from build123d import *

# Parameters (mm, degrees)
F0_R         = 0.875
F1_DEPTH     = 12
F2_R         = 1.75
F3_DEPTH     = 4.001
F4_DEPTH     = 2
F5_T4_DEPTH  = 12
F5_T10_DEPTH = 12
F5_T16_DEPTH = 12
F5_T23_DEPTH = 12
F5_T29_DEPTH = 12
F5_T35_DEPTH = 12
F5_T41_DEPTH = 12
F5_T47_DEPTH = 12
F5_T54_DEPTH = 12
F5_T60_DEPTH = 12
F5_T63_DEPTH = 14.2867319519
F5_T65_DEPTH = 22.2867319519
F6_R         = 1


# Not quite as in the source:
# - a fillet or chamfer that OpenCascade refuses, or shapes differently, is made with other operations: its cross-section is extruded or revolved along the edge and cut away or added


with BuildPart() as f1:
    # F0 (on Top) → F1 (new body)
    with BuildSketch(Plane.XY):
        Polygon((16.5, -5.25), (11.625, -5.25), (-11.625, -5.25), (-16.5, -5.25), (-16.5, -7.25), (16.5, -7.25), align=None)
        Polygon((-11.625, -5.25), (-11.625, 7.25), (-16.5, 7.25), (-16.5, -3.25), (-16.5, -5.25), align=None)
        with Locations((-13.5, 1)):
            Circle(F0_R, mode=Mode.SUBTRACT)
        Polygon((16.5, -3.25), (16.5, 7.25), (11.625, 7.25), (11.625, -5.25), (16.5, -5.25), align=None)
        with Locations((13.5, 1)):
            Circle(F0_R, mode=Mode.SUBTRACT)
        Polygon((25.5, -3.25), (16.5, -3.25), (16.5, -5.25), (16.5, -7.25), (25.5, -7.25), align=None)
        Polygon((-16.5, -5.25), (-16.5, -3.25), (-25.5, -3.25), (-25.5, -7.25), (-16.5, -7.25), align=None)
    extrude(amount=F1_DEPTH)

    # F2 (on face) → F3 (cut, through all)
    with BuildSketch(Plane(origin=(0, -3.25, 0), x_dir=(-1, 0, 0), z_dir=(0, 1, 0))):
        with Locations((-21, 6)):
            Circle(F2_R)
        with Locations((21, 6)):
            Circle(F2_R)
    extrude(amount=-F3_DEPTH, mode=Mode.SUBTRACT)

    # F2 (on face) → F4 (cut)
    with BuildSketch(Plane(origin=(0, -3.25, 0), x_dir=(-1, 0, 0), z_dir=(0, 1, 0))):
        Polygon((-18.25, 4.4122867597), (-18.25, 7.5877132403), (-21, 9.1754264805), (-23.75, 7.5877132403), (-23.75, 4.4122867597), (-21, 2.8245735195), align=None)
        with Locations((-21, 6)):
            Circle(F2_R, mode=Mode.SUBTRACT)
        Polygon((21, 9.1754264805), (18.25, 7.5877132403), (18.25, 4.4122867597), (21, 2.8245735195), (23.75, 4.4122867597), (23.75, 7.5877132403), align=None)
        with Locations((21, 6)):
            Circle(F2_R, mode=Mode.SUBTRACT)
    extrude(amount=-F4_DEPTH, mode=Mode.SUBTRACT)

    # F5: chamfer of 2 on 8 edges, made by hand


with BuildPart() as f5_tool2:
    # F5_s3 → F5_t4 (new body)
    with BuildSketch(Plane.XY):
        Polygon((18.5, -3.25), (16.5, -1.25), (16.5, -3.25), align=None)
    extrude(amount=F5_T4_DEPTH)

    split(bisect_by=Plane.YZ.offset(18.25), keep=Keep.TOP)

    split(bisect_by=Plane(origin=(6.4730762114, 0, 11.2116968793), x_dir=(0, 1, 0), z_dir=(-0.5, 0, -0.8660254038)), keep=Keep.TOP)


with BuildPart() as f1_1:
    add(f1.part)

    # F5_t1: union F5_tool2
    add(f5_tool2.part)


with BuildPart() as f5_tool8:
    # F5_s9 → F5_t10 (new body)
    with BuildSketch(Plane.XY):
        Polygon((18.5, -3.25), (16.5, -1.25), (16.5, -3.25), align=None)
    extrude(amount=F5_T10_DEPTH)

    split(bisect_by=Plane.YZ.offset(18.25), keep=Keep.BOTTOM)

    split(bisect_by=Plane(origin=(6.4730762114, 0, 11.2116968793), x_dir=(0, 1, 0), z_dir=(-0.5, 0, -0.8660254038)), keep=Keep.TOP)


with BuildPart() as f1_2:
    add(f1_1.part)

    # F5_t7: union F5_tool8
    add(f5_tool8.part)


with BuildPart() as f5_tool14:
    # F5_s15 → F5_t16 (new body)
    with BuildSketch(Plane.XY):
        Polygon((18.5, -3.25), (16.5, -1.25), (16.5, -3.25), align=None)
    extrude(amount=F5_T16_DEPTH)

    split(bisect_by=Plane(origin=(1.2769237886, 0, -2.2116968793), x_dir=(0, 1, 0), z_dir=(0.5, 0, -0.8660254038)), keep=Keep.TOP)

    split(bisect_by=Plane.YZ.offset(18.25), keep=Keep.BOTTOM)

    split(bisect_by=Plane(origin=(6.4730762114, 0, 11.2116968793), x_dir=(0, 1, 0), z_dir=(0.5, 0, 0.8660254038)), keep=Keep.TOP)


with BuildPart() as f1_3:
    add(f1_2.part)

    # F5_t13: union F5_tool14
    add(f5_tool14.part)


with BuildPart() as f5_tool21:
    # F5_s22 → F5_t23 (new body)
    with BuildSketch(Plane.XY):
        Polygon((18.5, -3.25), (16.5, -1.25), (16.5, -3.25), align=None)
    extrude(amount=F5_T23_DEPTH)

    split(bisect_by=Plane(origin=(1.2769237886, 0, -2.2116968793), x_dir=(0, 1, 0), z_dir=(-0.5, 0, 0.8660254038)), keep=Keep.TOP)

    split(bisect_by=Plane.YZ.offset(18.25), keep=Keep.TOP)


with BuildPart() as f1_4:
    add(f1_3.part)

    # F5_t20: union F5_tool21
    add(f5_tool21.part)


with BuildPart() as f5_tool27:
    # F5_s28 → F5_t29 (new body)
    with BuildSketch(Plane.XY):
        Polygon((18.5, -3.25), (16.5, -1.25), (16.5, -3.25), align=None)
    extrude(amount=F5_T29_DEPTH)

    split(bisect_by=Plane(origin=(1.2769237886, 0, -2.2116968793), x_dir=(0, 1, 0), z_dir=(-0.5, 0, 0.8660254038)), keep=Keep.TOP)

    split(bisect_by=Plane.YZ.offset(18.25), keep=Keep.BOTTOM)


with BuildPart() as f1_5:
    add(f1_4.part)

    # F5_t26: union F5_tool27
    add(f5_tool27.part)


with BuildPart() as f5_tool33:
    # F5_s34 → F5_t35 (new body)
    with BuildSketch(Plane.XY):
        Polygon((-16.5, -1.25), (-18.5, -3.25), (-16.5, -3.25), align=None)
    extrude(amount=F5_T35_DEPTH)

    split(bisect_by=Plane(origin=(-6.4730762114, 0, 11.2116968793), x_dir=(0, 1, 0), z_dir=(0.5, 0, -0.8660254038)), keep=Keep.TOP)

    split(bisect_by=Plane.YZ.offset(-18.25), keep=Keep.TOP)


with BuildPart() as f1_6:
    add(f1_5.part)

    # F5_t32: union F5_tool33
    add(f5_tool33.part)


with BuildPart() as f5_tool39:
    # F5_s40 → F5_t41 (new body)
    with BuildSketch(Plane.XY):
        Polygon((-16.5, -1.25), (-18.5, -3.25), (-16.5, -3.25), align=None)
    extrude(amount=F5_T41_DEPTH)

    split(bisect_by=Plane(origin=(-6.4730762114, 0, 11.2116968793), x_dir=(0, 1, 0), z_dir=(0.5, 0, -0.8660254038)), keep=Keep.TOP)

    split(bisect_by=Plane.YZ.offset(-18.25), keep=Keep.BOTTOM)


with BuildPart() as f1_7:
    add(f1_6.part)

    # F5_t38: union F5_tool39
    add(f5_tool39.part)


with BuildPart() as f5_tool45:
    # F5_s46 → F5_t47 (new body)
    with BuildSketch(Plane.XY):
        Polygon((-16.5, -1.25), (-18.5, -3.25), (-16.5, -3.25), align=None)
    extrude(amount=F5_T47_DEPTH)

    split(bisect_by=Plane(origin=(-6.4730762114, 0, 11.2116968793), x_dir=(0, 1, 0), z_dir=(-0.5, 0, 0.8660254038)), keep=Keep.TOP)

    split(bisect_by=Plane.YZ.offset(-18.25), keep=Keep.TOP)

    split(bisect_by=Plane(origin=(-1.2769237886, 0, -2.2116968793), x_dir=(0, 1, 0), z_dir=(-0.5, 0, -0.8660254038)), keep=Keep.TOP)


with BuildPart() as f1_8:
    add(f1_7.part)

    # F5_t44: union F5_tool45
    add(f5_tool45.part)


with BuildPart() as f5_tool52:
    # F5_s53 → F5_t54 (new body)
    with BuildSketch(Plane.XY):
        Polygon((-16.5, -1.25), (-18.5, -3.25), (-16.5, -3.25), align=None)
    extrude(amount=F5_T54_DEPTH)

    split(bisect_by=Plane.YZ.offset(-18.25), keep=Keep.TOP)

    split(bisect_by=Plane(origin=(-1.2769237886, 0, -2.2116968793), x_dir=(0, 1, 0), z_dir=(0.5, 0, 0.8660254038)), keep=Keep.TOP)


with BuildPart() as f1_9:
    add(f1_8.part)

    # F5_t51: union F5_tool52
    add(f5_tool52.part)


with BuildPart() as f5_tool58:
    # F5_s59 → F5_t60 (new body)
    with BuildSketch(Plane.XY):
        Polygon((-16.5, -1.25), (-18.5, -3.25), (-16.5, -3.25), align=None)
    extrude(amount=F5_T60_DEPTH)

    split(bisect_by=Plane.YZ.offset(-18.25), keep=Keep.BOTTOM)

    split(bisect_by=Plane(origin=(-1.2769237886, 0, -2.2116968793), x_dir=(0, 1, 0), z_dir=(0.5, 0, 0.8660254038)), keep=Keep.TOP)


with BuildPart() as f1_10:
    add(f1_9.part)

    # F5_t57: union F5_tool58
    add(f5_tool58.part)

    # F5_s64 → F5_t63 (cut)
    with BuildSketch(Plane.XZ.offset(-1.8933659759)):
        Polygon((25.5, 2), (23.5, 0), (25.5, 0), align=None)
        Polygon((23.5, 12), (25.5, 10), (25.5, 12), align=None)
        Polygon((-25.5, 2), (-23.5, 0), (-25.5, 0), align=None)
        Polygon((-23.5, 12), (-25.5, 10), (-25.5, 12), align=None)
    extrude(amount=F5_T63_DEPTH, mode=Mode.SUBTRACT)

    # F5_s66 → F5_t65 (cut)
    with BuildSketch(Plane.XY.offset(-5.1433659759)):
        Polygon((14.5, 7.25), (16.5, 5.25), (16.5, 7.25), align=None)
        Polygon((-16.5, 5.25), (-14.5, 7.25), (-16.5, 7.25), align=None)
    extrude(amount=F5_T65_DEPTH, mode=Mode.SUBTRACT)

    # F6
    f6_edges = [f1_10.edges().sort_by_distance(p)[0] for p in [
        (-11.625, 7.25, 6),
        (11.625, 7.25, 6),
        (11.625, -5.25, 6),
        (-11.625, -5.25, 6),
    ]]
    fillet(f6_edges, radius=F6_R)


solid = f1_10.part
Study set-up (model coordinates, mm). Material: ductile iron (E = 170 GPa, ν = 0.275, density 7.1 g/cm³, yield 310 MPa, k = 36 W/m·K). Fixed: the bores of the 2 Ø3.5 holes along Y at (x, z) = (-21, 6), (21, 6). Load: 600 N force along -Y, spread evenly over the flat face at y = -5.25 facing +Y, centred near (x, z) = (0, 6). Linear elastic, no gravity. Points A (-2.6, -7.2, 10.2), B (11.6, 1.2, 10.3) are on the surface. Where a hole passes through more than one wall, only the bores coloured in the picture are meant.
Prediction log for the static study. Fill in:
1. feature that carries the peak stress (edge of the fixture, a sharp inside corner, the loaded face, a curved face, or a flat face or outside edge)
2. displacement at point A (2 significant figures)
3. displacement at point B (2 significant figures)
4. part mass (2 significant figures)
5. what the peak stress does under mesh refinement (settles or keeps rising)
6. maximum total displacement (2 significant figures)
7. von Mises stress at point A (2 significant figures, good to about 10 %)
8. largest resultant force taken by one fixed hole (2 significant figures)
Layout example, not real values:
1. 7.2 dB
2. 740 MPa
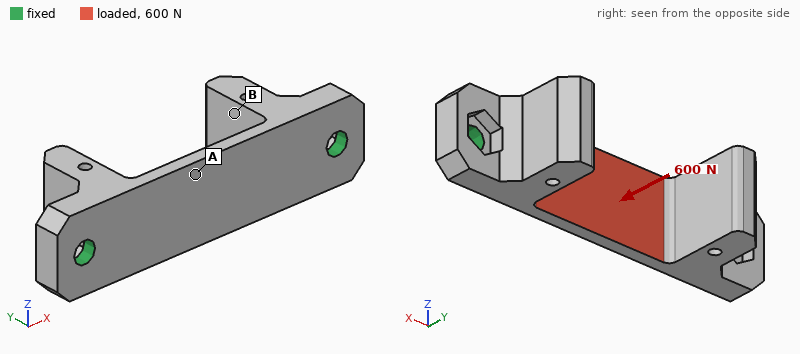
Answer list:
1. edge of the fixture
2. 54 µm
3. 29 µm
4. 20 g
5. keeps rising
6. 58 µm
7. 120 MPa
8. 360 N
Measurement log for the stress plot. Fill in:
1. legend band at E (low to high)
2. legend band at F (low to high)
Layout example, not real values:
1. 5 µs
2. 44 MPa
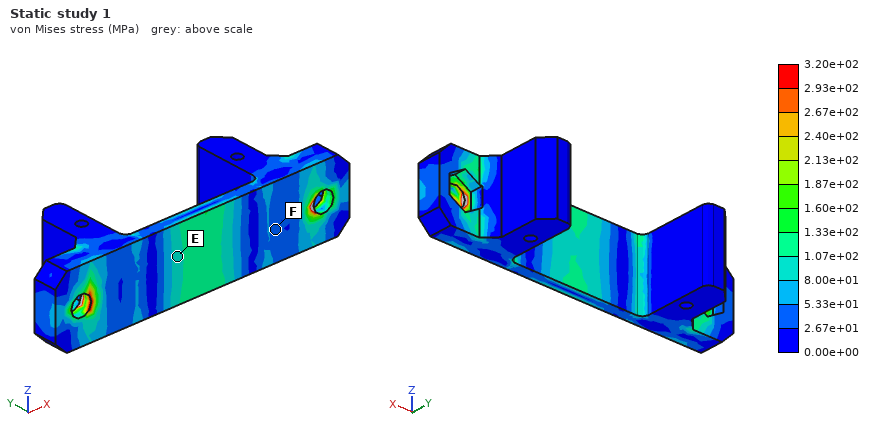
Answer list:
1. 8.00e+01 to 1.07e+02 MPa
2. 2.67e+01 to 5.33e+01 MPa
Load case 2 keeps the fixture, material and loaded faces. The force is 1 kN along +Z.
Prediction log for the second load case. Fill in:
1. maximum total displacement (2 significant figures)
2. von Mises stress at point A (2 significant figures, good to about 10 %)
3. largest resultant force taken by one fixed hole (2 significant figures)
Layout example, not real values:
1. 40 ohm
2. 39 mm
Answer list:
1. 17 µm
2. 69 MPa
3. 500 N
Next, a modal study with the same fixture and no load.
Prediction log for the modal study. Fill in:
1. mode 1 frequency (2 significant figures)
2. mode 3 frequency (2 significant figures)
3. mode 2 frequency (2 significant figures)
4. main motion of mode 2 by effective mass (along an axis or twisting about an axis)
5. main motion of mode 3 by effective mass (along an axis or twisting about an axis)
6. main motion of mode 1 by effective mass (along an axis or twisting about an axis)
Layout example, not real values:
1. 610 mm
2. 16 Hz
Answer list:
1. 6500 Hz
2. 10 kHz
3. 9400 Hz
4. along X
5. along Z
6. along Y
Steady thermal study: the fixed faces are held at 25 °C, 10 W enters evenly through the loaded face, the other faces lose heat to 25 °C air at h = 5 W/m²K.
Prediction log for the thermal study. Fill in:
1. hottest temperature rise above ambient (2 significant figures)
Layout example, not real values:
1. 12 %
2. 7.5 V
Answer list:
1. 68 K
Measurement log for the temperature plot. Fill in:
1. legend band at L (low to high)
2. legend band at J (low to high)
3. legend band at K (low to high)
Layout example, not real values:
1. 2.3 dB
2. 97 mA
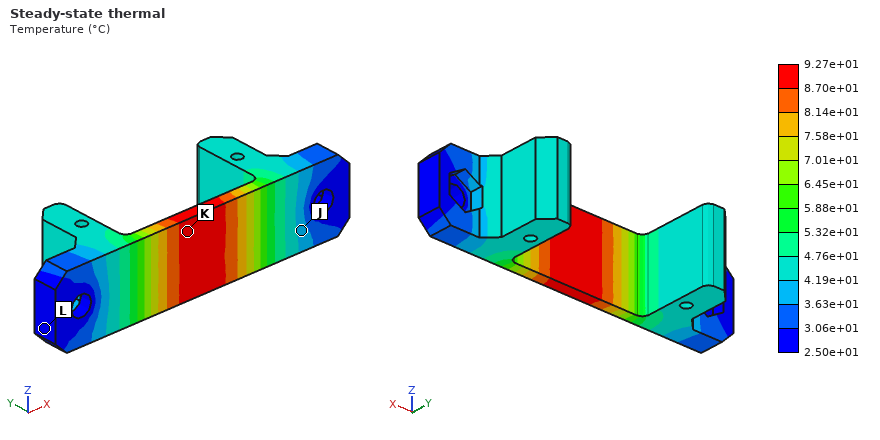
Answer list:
1. 2.50e+01 to 3.06e+01 °C
2. 3.63e+01 to 4.19e+01 °C
3. 8.70e+01 to 9.27e+01 °C
